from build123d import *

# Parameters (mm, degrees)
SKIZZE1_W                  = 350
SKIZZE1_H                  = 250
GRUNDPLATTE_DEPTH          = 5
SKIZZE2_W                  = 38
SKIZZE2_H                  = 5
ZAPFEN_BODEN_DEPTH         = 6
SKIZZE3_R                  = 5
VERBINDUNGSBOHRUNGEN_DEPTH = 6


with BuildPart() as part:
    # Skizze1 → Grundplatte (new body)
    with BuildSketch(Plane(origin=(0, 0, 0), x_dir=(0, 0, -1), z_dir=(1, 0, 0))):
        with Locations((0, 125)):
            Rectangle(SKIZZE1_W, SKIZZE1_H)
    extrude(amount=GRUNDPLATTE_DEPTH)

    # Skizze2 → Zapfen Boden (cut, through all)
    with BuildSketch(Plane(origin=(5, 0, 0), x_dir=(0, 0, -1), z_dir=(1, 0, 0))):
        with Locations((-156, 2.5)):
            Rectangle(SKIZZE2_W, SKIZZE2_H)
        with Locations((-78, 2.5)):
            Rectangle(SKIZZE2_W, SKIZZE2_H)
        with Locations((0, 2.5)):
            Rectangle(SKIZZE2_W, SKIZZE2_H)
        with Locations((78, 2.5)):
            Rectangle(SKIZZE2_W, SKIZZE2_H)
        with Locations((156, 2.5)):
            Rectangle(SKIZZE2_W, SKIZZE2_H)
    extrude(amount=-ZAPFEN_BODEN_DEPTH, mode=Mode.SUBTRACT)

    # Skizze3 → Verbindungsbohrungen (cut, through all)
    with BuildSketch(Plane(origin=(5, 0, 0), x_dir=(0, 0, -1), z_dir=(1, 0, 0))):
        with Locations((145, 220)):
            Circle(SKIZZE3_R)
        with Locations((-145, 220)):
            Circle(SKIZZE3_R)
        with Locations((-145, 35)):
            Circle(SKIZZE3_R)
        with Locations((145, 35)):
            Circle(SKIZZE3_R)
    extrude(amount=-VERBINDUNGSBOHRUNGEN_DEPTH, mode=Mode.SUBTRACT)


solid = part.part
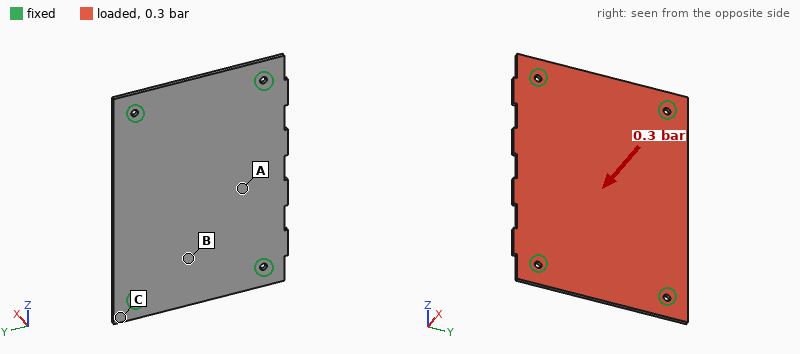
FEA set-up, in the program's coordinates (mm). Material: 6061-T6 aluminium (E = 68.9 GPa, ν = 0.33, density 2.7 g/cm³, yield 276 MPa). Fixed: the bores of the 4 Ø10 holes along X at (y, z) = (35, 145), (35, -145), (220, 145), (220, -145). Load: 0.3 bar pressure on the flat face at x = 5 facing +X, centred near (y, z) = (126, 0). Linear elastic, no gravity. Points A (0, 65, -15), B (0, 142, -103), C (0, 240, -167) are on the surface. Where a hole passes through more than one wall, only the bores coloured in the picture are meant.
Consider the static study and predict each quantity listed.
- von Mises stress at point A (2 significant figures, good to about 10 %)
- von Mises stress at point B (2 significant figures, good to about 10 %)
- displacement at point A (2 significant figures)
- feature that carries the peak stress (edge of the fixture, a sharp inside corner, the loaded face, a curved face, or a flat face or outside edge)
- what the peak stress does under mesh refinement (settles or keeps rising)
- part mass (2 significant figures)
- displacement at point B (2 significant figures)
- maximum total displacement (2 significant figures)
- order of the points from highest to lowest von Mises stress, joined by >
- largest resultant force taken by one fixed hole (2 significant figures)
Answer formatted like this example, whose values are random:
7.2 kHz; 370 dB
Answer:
26 MPa; 14 MPa; 0.98 mm; edge of the fixture; keeps rising; 1.2 kg; 0.48 mm; 1.1 mm; A > B > C; 650 N
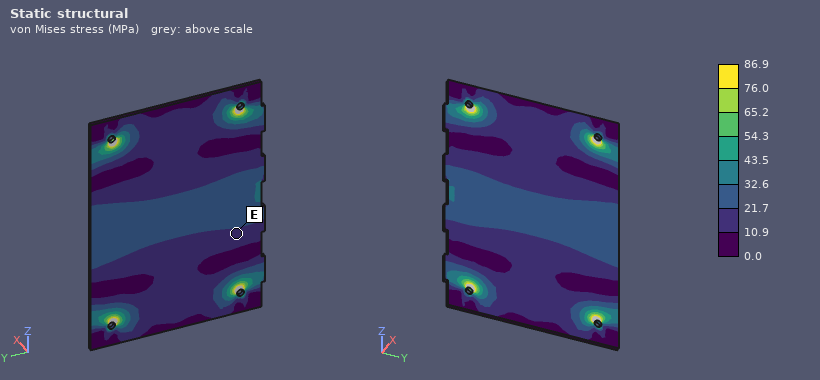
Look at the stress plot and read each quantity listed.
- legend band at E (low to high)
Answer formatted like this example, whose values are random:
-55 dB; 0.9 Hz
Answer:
10.9 to 21.7 MPa
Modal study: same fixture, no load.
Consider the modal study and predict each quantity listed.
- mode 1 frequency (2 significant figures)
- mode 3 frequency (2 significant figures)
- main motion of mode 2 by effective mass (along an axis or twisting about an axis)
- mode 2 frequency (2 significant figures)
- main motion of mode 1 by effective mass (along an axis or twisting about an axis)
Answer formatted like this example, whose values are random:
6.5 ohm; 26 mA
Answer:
270 Hz; 620 Hz; twisting about Z; 390 Hz; along X
